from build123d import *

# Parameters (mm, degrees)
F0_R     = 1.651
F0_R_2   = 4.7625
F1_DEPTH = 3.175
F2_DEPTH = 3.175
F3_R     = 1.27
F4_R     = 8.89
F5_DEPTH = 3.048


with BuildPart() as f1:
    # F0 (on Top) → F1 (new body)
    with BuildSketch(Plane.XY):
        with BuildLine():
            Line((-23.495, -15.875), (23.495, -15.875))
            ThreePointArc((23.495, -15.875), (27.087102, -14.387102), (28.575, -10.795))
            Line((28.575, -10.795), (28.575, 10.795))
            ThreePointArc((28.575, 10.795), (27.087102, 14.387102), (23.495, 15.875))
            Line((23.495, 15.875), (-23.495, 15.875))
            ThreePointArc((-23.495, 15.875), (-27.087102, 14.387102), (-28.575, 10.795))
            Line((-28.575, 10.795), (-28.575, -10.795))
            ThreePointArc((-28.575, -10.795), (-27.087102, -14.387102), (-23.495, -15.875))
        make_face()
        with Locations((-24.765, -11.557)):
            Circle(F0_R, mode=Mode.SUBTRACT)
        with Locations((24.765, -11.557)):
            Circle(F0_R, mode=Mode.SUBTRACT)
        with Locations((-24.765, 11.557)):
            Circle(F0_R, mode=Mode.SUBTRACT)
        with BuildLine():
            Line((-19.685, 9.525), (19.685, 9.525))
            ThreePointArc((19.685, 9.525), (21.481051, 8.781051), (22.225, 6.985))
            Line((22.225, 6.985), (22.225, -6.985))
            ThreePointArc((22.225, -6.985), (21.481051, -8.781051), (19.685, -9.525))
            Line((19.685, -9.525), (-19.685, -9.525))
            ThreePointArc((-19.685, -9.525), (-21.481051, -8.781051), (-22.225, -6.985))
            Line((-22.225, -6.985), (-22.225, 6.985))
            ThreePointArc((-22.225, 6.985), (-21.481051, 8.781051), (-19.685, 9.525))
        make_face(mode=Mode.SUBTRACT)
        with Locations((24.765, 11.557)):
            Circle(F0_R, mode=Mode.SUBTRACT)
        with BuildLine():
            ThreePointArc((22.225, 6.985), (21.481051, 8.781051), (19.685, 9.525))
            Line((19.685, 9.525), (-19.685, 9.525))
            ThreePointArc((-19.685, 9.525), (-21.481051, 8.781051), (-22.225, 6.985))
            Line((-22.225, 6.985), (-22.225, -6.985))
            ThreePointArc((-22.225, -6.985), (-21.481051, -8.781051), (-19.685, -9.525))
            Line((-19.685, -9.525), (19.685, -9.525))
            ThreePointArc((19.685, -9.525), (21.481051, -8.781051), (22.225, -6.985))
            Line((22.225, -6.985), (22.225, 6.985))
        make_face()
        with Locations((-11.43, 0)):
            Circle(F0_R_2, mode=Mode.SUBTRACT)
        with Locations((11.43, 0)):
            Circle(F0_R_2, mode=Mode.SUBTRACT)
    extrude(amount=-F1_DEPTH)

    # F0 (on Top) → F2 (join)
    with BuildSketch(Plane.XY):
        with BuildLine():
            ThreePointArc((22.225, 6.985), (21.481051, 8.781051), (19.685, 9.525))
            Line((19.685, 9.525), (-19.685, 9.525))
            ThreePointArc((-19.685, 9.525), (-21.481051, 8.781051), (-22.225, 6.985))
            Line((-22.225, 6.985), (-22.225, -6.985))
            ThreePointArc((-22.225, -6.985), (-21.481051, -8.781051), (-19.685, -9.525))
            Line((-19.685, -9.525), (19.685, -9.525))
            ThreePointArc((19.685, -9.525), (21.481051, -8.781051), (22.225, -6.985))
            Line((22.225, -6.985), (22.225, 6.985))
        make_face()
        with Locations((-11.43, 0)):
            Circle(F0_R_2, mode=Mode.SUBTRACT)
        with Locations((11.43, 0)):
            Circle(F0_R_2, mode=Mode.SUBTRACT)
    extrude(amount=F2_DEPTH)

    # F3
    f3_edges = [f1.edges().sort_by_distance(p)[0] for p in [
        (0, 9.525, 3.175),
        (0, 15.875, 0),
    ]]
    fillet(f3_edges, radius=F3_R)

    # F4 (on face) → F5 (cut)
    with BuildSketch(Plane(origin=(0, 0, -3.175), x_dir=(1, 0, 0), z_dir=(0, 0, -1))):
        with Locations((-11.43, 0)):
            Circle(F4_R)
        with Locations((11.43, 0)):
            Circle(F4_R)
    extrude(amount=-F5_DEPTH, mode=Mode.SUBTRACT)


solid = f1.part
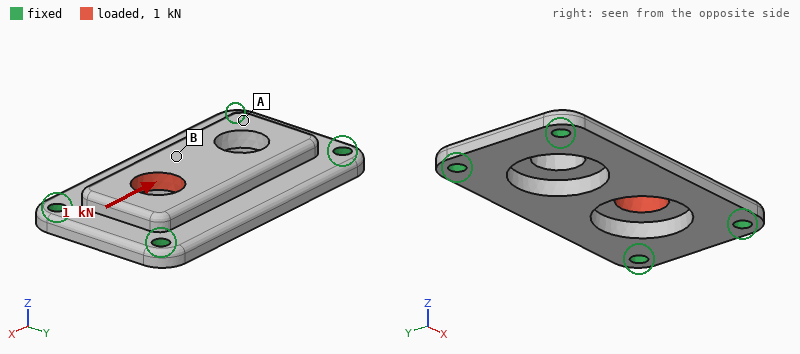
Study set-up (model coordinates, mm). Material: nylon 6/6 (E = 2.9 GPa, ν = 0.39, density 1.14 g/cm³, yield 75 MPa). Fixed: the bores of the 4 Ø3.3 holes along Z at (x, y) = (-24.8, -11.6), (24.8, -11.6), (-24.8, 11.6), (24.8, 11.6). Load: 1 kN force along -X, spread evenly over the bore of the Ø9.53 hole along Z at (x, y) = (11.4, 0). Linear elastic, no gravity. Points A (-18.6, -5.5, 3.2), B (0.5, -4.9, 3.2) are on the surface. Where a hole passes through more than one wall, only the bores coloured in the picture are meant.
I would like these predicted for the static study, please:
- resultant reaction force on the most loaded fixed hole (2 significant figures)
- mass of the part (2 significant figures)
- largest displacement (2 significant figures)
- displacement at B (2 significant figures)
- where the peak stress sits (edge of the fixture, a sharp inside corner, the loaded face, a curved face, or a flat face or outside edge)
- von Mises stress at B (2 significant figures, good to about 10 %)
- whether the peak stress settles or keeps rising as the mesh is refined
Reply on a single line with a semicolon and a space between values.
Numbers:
310 N; 7.0 g; 0.15 mm; 0.10 mm; edge of the fixture; 9.8 MPa; keeps rising
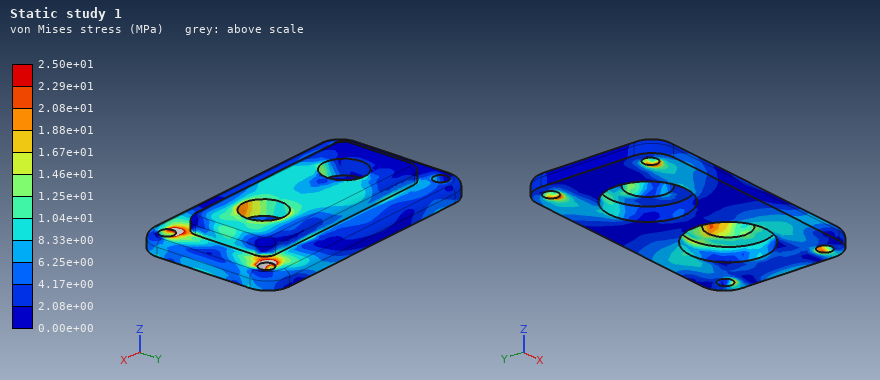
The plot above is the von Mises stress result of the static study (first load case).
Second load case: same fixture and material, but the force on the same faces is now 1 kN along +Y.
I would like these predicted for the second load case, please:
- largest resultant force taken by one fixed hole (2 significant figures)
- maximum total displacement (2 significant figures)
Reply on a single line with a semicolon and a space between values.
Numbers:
430 N; 0.19 mm
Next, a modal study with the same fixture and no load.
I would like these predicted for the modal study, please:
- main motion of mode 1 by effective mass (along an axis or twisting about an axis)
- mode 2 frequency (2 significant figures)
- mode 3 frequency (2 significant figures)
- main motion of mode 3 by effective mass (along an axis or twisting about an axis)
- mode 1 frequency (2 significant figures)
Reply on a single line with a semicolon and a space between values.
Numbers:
along Z; 3300 Hz; 6000 Hz; along Y; 2500 Hz
